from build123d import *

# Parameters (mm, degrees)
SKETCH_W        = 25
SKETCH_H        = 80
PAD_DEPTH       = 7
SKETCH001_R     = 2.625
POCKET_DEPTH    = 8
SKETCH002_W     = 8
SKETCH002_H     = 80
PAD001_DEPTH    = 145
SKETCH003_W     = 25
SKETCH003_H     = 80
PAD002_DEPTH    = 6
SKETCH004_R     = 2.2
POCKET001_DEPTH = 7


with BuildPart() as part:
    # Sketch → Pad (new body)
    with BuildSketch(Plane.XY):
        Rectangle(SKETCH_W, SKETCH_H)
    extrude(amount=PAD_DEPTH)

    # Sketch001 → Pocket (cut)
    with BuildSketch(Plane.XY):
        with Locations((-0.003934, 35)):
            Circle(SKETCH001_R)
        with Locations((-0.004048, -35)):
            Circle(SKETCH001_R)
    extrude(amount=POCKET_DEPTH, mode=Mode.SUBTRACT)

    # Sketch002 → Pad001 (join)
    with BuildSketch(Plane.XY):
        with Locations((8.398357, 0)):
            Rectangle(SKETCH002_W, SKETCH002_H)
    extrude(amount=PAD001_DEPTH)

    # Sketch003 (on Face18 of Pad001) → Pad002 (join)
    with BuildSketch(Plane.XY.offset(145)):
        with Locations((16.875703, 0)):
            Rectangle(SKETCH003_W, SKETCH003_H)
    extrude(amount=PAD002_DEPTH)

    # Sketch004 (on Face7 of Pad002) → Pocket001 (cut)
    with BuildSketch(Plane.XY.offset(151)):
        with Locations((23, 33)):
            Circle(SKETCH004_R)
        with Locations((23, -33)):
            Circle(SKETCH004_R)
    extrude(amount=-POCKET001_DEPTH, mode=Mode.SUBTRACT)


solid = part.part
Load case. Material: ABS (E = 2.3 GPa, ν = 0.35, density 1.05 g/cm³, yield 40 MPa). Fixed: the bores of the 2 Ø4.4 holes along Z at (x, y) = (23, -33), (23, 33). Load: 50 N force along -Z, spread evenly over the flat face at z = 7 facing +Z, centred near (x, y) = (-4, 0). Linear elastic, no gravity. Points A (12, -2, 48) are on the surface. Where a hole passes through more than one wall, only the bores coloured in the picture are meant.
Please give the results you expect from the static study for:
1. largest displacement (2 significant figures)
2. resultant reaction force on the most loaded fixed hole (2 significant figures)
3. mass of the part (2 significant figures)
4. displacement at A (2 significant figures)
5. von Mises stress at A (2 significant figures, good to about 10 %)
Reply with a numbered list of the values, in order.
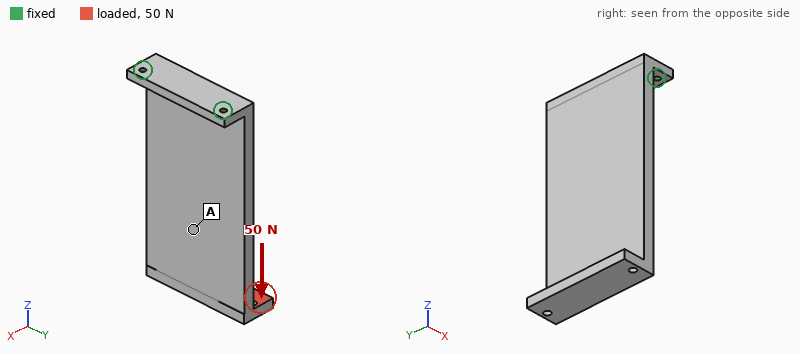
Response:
1. 1.9 mm
2. 25 N
3. 120 g
4. 1.1 mm
5. 0.60 MPa
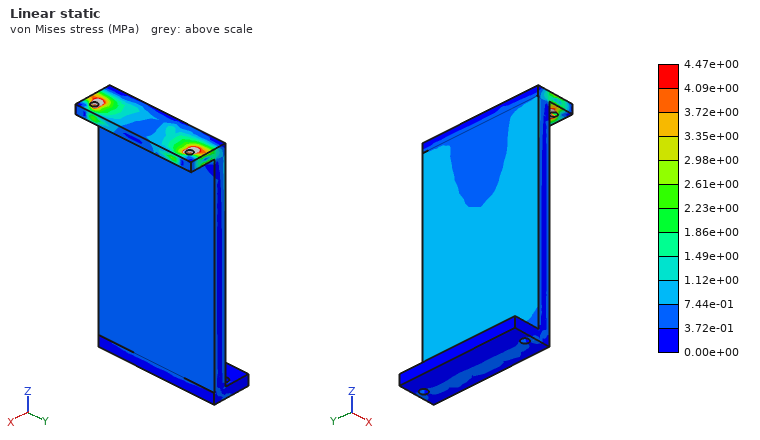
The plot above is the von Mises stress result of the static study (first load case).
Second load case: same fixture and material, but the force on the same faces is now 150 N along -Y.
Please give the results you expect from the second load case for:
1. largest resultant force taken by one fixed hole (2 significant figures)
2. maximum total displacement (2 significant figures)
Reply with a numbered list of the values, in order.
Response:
1. 340 N
2. 1.5 mm
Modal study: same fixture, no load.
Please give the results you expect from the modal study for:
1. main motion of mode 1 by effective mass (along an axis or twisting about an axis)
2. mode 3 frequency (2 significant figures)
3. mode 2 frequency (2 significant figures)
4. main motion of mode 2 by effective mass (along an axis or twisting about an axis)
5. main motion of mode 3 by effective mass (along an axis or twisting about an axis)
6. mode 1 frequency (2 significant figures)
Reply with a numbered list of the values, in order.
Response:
1. along X
2. 300 Hz
3. 250 Hz
4. along Y
5. along Y
6. 50 Hz
